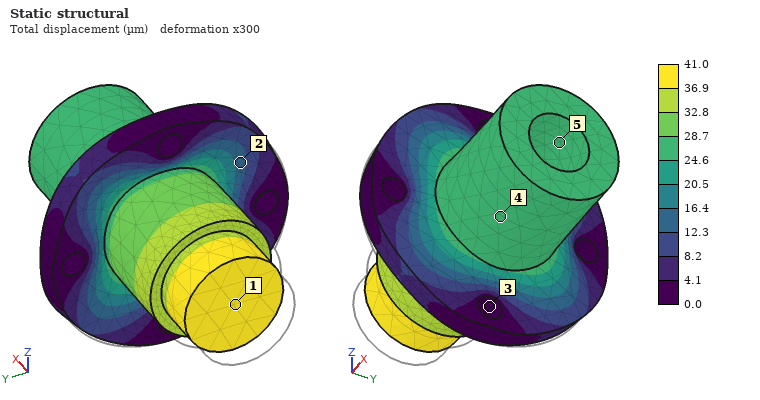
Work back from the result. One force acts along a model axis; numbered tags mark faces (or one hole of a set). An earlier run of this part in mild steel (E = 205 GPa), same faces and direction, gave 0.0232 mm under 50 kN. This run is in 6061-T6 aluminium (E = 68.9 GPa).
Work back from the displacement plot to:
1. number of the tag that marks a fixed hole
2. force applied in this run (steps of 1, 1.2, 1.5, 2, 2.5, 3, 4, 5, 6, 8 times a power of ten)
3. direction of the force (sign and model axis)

3
30 kN
+X
